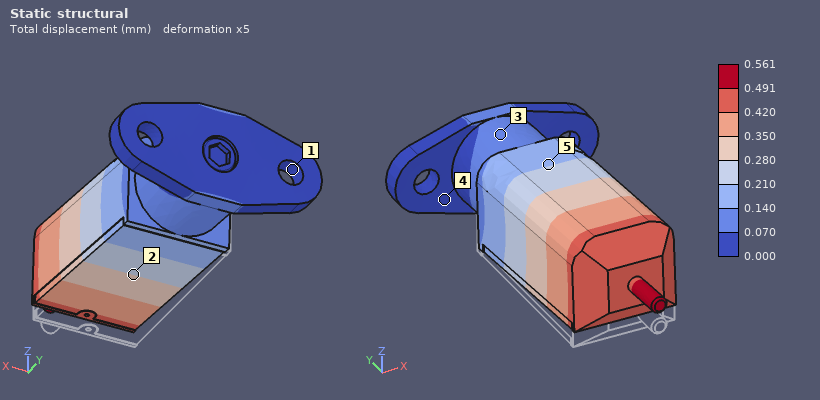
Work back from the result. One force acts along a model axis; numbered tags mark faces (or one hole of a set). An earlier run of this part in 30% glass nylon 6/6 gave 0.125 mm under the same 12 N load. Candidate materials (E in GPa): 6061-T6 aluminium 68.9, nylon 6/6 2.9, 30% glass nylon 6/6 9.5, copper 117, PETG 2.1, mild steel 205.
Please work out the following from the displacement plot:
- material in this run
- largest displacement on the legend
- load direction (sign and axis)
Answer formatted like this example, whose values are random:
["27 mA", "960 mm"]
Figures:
["PETG", "0.561 mm", "+Z"]
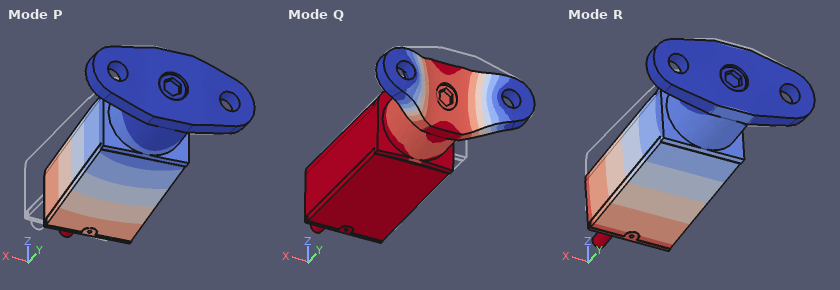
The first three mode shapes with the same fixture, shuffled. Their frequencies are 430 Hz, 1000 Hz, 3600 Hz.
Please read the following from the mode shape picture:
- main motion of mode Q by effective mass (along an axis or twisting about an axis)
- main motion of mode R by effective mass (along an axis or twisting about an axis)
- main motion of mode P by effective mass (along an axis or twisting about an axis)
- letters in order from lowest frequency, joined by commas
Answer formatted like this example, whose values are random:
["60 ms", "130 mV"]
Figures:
["along Y", "along Z", "along X", "R, P, Q"]
